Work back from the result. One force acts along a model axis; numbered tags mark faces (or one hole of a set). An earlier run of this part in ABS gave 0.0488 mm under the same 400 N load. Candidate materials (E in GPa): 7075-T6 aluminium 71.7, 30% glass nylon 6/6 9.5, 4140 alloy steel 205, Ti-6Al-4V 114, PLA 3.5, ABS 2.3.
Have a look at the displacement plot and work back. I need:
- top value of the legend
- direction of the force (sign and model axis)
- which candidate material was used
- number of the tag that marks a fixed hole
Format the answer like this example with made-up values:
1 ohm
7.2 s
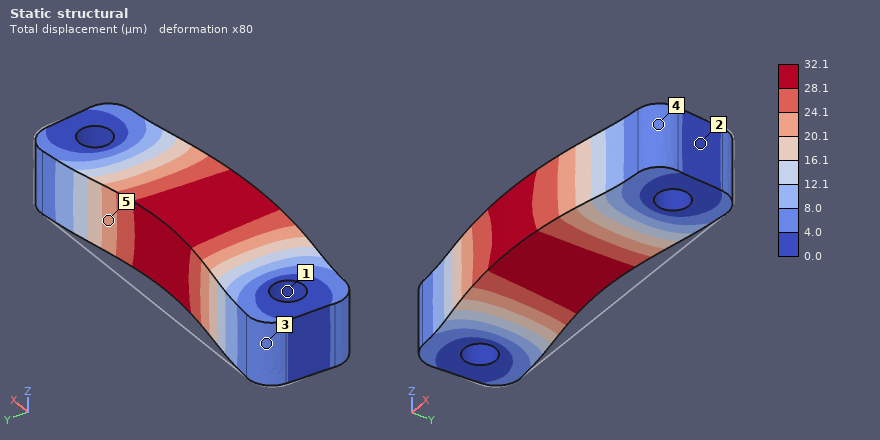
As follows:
32.1 µm
-Y
PLA
1
